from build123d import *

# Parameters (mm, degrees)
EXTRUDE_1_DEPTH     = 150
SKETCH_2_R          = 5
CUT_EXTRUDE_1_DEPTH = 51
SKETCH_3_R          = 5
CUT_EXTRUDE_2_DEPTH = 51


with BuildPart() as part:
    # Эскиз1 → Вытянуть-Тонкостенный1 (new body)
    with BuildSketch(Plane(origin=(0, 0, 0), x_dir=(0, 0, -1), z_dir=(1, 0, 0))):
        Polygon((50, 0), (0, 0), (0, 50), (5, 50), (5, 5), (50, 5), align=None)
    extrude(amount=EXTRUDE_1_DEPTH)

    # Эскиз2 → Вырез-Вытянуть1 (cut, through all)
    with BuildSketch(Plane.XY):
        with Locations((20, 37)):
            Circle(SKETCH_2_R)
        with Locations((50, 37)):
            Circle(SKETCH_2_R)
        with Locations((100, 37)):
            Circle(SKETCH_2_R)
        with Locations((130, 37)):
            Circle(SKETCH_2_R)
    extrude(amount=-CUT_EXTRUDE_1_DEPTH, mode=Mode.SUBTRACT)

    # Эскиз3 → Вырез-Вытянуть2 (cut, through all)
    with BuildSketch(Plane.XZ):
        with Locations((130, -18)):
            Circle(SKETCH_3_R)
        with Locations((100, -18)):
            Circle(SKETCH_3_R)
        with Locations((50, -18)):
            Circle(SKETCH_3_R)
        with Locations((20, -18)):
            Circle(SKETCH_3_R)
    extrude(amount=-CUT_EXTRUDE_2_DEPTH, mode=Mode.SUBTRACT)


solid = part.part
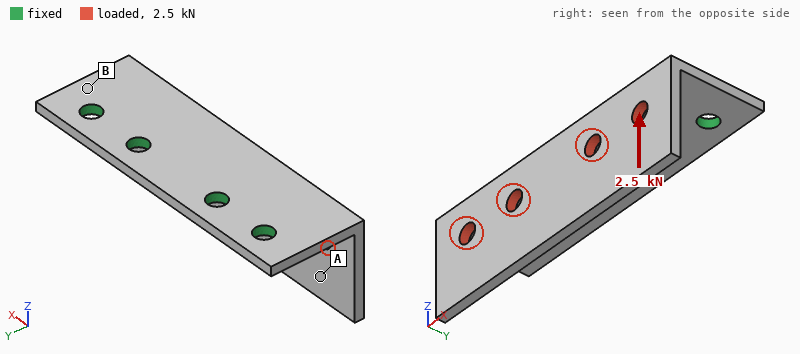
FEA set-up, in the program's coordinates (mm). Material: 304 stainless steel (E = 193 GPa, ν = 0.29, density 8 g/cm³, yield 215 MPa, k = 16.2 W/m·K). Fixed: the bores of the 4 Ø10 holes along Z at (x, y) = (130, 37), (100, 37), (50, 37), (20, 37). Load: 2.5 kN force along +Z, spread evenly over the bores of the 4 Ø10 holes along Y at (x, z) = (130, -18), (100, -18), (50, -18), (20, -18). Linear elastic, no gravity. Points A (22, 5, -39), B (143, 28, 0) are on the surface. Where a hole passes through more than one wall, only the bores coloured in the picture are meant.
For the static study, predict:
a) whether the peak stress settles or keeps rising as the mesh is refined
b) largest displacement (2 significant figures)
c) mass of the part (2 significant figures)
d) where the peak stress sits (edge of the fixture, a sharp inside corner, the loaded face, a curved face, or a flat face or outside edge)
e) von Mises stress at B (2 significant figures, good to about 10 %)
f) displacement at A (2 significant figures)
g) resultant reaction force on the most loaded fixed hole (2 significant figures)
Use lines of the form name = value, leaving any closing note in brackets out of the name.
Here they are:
whether the peak stress settles or keeps rising as the mesh is refined = keeps rising
largest displacement = 0.23 mm
mass of the part = 540 g
where the peak stress sits = edge of the fixture
von Mises stress at B = 78 MPa
displacement at A = 0.17 mm
resultant reaction force on the most loaded fixed hole = 650 N
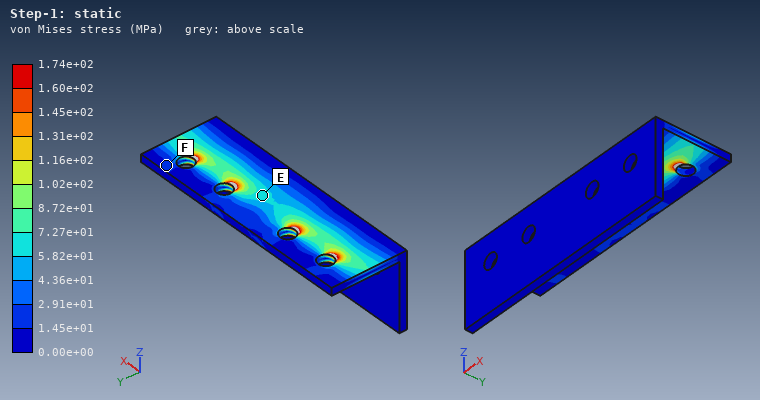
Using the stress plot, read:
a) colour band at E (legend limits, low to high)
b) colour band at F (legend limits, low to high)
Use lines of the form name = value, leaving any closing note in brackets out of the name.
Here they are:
colour band at E = 5.82e+01 to 7.27e+01 MPa
colour band at F = 1.45e+01 to 2.91e+01 MPa
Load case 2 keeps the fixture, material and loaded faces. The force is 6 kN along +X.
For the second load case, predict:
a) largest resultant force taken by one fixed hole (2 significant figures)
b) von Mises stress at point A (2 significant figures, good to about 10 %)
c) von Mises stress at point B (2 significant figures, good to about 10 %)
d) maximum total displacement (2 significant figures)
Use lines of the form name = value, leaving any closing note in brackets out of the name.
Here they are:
largest resultant force taken by one fixed hole = 2.1 kN
von Mises stress at point A = 11 MPa
von Mises stress at point B = 65 MPa
maximum total displacement = 0.13 mm
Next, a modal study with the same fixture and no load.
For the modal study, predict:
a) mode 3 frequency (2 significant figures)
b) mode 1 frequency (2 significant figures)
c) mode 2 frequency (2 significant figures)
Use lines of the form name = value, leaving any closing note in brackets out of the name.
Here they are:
mode 3 frequency = 2300 Hz
mode 1 frequency = 830 Hz
mode 2 frequency = 1300 Hz
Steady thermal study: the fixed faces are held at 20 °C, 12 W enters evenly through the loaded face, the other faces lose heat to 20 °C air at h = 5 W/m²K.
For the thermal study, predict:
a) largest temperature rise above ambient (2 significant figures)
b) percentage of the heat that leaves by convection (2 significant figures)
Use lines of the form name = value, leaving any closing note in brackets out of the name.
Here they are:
largest temperature rise above ambient = 43 K
percentage of the heat that leaves by convection = 27 %
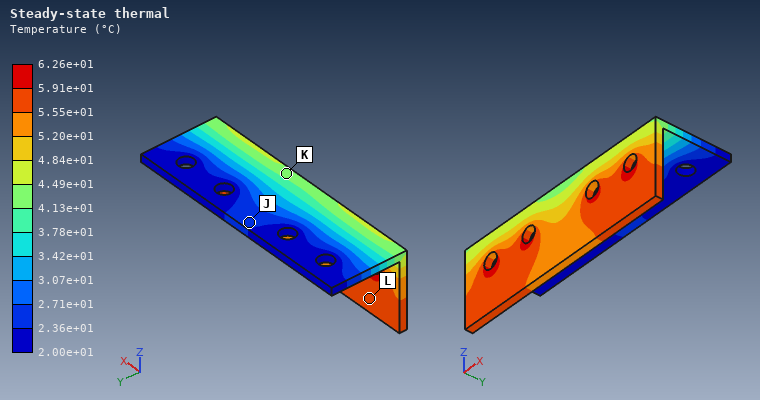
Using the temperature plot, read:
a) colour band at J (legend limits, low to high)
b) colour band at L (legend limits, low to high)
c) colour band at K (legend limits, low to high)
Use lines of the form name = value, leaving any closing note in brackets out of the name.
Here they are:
colour band at J = 2.36e+01 to 2.71e+01 °C
colour band at L = 5.55e+01 to 5.91e+01 °C
colour band at K = 4.13e+01 to 4.49e+01 °C
